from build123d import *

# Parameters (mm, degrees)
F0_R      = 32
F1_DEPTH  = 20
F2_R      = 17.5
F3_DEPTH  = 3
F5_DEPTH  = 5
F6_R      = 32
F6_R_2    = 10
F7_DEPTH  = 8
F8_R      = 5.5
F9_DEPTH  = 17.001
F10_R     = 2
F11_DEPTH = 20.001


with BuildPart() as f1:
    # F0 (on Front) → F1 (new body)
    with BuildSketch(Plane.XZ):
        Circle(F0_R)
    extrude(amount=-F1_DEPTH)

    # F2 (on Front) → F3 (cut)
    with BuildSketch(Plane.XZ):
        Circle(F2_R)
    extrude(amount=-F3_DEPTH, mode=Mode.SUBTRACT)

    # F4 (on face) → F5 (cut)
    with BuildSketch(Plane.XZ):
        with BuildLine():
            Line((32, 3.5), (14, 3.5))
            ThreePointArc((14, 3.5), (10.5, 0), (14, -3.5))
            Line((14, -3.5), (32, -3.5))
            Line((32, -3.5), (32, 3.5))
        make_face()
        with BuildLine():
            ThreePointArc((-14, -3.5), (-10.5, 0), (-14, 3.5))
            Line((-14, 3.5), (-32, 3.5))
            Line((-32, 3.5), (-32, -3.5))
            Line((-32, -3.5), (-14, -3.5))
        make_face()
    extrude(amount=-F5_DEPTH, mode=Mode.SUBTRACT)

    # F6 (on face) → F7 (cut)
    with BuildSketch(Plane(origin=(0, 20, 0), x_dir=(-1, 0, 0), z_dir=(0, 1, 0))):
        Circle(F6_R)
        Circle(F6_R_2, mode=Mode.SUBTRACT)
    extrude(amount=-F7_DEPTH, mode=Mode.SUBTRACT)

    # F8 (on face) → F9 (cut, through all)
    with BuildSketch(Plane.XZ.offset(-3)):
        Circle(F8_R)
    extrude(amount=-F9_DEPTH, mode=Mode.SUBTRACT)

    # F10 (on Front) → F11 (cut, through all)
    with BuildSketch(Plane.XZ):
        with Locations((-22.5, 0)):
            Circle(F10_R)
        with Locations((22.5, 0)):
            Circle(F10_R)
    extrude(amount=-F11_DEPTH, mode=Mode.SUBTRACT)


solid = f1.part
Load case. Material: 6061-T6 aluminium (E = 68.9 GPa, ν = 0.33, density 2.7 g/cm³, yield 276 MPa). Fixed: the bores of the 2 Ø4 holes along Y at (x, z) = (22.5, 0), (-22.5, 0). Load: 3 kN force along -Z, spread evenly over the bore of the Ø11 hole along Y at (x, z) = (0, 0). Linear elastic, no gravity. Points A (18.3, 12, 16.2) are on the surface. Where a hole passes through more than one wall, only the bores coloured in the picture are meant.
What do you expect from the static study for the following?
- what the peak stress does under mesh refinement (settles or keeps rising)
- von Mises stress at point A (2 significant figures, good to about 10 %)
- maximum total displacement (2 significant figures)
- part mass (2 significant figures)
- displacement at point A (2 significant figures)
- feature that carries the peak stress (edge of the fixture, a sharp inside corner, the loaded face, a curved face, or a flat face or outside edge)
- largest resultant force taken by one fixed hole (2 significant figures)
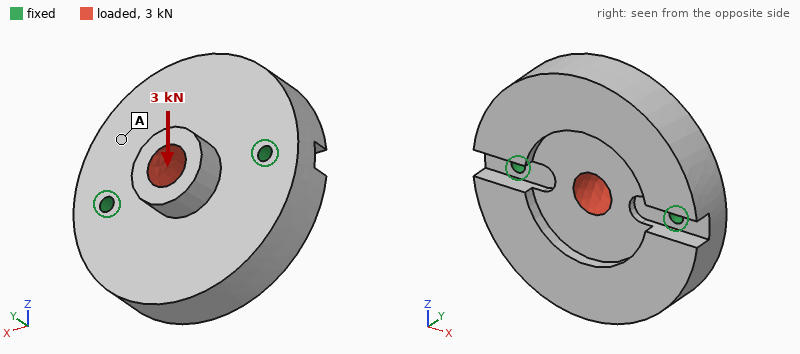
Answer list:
keeps rising
5.4 MPa
18 µm
95 g
8.3 µm
edge of the fixture
1.5 kN
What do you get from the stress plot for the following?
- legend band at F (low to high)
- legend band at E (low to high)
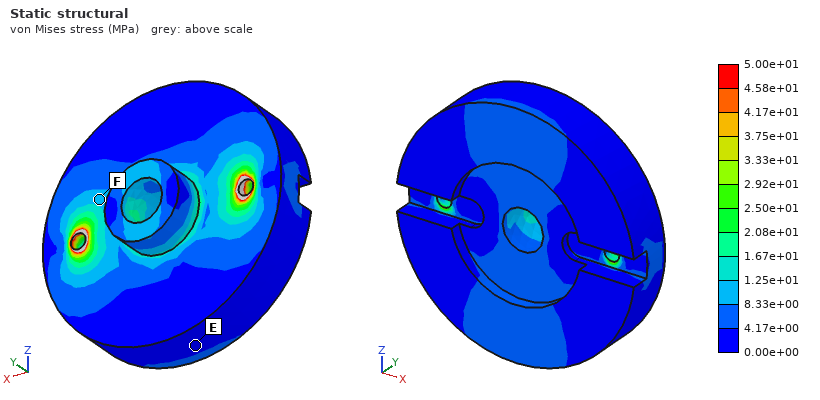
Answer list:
8.33e+00 to 1.25e+01 MPa
0.00e+00 to 4.17e+00 MPa
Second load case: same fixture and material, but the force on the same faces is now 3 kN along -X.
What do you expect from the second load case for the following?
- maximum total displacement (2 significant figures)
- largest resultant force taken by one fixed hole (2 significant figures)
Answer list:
7.2 µm
1.5 kN
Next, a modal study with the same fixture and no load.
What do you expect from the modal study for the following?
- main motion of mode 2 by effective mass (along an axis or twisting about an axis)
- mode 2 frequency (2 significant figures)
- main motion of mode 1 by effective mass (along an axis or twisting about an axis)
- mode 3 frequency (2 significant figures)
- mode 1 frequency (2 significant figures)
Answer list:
along Y
6500 Hz
twisting about X
13 kHz
4100 Hz
